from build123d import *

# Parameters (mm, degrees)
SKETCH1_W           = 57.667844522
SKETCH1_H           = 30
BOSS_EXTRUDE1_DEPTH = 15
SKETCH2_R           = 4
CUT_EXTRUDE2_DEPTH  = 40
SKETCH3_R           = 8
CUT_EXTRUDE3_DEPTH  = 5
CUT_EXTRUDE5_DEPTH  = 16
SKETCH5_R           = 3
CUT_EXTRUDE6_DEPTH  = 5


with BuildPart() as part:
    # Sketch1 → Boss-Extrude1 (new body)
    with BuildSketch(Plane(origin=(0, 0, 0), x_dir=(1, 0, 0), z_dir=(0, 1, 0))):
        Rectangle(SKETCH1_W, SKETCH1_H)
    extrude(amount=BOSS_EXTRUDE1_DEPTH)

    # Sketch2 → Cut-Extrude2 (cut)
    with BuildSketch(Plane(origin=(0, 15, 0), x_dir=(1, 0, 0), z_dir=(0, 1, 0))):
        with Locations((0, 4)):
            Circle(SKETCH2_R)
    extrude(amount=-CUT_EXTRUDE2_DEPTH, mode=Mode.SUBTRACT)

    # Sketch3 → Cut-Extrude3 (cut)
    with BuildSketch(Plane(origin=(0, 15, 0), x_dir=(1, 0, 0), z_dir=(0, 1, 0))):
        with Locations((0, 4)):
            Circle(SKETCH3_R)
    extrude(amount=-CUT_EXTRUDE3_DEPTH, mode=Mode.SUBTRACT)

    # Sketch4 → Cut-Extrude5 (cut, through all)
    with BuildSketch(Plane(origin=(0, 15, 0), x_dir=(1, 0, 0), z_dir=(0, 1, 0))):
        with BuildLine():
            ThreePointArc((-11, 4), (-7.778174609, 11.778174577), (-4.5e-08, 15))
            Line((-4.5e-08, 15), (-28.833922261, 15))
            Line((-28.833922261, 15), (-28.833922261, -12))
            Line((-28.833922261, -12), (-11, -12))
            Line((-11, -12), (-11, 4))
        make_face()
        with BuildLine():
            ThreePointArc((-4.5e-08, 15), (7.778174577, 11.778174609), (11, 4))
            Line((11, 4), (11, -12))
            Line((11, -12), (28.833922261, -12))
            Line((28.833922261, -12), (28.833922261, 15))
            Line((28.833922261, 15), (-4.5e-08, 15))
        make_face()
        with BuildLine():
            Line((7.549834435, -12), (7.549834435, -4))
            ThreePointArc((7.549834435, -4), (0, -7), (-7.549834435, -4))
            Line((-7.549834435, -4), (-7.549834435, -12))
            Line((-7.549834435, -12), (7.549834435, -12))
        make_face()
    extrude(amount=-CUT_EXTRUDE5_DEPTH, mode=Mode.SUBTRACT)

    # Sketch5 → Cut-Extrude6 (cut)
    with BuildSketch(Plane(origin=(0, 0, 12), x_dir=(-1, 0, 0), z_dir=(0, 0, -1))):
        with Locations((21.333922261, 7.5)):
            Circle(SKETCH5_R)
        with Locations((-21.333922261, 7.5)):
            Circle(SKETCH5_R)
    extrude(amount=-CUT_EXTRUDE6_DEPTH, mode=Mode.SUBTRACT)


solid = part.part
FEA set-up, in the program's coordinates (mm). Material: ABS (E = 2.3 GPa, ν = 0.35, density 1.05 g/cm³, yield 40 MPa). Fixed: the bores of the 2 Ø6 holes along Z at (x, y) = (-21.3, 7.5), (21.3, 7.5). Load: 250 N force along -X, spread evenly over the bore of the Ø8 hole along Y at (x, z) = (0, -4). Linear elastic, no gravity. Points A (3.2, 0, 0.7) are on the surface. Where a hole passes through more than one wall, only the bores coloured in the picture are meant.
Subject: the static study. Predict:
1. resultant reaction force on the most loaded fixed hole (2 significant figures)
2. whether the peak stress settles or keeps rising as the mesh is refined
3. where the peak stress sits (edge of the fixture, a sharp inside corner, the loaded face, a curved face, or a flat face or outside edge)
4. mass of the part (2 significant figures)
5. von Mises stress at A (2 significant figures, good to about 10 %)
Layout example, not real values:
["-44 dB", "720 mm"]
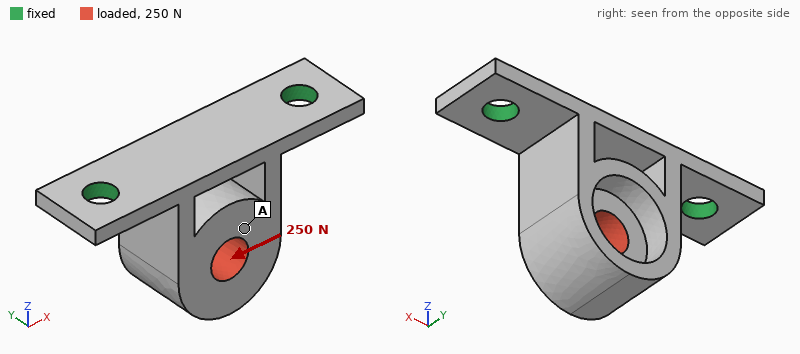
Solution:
["190 N", "keeps rising", "edge of the fixture", "8.1 g", "3.2 MPa"]
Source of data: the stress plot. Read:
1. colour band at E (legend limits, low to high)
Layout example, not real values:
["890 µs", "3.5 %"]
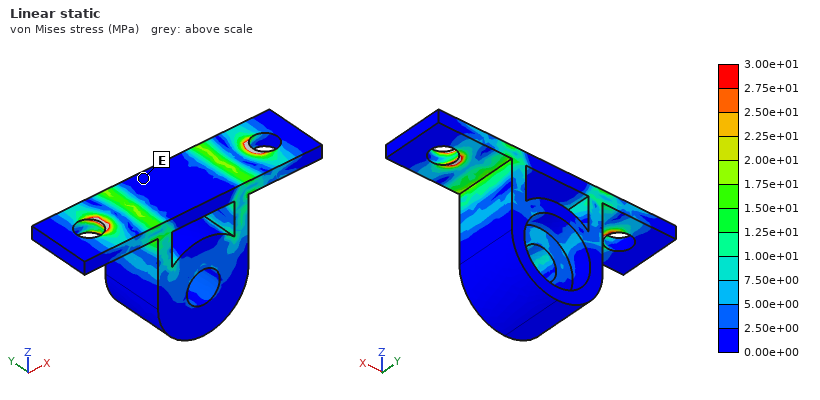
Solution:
["0.00e+00 to 2.50e+00 MPa"]
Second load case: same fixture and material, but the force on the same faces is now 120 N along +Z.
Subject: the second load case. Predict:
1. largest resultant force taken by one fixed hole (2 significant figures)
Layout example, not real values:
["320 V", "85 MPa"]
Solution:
["63 N"]
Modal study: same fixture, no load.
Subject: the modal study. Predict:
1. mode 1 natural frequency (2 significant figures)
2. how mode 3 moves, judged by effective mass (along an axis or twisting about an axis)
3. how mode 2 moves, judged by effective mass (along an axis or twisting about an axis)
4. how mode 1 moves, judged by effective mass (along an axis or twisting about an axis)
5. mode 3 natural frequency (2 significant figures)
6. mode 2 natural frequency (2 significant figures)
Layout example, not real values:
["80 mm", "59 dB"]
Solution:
["690 Hz", "along Z", "along X", "along Y", "2100 Hz", "1800 Hz"]
